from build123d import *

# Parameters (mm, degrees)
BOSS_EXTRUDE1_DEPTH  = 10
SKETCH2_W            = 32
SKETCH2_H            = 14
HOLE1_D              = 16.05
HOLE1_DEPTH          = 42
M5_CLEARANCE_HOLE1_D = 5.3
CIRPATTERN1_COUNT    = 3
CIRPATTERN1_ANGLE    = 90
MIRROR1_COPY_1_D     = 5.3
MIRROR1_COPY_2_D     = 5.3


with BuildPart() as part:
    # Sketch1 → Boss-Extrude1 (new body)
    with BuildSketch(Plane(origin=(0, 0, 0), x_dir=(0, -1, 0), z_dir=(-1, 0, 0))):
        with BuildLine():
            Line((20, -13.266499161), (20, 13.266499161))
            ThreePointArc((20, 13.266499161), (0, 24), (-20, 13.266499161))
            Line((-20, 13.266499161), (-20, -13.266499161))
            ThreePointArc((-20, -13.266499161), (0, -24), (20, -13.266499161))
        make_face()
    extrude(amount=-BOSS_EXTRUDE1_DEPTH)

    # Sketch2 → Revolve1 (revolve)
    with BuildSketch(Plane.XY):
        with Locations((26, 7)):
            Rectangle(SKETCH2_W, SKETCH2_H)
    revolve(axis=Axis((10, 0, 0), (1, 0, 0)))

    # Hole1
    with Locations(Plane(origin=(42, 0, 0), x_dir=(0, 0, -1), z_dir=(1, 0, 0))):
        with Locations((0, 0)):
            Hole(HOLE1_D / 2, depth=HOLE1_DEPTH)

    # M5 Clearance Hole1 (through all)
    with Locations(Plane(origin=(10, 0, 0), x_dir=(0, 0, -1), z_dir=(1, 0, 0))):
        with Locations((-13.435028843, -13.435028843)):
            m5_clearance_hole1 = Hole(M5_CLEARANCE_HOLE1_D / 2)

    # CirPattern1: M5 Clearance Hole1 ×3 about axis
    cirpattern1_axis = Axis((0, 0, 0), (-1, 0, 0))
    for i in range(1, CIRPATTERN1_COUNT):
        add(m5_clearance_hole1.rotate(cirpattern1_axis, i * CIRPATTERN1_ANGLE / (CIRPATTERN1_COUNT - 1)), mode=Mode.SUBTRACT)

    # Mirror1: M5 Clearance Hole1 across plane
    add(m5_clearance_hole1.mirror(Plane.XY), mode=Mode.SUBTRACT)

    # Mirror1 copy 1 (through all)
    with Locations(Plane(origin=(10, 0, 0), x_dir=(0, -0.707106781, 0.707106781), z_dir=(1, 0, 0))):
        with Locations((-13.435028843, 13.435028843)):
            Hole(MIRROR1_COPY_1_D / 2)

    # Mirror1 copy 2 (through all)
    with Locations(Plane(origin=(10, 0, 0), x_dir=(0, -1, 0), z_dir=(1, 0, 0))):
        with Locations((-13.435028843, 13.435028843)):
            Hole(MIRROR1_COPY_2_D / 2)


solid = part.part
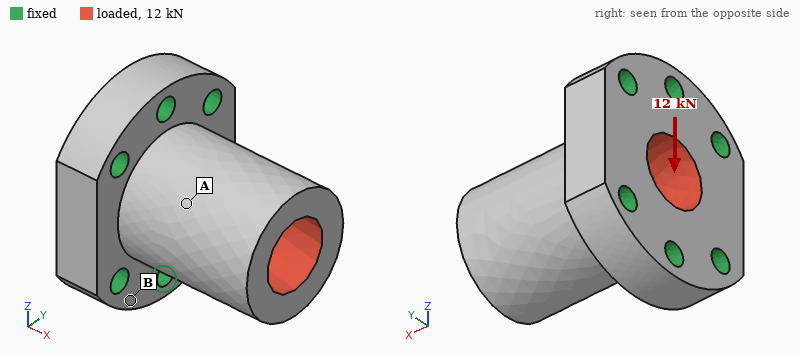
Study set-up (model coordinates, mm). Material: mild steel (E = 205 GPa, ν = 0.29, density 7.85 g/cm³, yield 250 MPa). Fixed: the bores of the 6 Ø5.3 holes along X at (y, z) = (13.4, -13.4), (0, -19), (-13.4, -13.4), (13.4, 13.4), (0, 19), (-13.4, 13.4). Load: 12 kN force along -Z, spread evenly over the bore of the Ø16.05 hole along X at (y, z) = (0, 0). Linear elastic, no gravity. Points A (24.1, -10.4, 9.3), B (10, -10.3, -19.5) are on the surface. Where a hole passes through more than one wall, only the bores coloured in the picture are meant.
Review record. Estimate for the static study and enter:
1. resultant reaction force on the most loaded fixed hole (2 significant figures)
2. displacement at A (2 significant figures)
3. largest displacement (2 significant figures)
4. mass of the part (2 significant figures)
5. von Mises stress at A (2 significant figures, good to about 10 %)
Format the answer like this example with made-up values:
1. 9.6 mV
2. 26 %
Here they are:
1. 3.7 kN
2. 11 µm
3. 22 µm
4. 210 g
5. 27 MPa
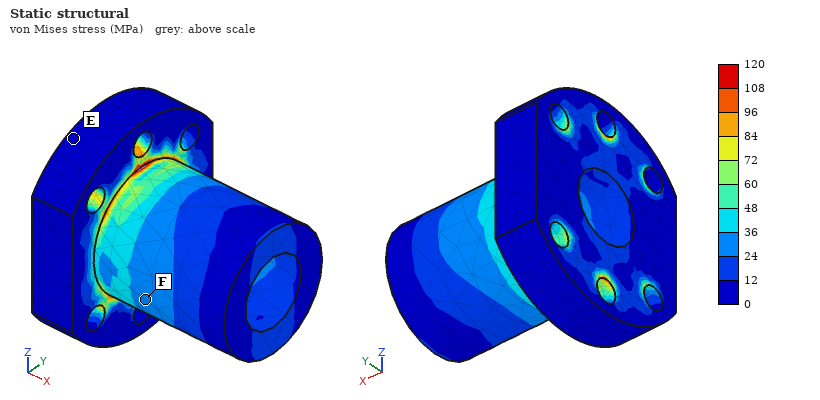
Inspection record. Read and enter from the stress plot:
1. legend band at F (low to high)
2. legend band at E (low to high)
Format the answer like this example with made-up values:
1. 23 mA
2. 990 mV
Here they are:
1. 24 to 36 MPa
2. 0 to 12 MPa
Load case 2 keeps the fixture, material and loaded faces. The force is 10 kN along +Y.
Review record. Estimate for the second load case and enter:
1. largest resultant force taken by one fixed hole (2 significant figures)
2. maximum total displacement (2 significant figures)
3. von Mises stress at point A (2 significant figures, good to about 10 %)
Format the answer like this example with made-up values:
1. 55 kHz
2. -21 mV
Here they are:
1. 3.7 kN
2. 21 µm
3. 22 MPa
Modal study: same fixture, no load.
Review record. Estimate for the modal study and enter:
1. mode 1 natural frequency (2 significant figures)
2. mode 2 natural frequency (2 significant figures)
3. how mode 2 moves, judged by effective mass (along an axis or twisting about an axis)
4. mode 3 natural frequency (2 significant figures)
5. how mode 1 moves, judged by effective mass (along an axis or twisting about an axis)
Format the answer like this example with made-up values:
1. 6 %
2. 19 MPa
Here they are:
1. 11 kHz
2. 12 kHz
3. along Z
4. 22 kHz
5. along Y
